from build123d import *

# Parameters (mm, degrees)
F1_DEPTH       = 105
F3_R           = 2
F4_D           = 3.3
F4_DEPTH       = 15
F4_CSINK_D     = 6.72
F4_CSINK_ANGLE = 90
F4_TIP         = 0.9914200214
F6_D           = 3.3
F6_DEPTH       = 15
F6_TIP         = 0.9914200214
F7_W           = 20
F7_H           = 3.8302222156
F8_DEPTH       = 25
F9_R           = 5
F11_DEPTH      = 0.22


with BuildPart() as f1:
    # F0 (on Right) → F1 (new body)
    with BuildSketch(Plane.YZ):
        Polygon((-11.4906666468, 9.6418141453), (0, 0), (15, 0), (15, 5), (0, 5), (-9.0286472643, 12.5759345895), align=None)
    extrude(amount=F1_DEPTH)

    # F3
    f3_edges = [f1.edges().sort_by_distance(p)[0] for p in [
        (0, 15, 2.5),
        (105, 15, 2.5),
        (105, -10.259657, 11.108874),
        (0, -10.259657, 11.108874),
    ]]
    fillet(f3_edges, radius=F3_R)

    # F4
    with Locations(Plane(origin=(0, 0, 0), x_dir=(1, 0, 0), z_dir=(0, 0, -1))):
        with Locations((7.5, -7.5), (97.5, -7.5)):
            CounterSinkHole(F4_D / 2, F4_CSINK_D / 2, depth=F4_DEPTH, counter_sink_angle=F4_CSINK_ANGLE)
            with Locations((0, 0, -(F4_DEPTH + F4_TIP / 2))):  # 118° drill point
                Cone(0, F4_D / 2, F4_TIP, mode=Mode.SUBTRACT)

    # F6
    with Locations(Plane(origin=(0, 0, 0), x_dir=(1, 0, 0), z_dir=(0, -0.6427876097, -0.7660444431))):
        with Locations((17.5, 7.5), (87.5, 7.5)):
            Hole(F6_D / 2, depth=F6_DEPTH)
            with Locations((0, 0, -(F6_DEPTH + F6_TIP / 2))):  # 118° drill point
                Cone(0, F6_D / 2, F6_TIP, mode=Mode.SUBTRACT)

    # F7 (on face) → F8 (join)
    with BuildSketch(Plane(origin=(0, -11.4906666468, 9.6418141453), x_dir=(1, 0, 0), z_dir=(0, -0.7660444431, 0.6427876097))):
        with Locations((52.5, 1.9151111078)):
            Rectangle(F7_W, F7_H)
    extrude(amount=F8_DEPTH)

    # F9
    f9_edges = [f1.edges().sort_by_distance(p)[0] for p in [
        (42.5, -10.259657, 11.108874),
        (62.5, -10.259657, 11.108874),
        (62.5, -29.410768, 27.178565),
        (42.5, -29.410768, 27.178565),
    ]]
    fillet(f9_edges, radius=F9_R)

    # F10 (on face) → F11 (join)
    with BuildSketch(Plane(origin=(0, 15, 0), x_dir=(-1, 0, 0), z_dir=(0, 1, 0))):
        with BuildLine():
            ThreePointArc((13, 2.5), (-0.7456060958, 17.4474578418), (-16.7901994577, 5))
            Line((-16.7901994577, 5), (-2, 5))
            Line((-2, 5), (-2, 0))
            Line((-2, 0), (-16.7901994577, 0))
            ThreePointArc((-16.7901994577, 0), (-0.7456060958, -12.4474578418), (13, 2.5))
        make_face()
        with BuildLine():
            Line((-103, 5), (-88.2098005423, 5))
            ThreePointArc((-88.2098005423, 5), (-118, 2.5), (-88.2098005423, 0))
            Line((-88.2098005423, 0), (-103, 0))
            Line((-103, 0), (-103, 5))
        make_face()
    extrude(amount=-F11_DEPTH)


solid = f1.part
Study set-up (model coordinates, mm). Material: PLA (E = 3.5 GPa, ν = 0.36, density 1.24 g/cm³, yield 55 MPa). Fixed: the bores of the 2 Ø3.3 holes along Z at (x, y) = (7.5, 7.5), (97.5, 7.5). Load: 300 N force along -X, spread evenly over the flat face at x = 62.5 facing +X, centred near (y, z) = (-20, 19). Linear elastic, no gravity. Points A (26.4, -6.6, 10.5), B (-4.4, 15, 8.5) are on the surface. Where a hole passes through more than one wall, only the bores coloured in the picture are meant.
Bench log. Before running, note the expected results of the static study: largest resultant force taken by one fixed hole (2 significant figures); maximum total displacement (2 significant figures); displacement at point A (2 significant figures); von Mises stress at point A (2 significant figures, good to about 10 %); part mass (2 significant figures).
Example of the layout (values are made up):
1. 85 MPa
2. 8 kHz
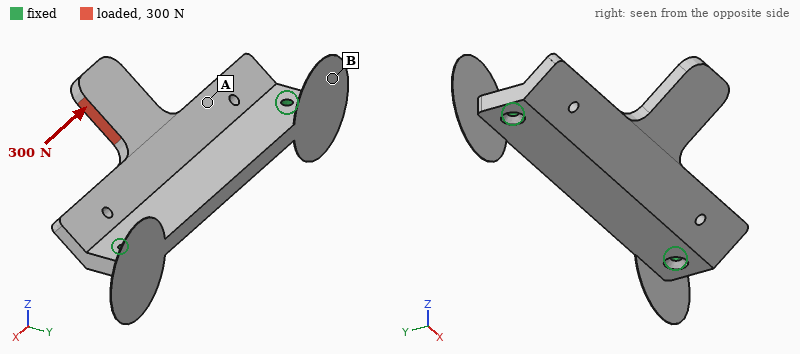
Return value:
1. 180 N
2. 0.30 mm
3. 0.11 mm
4. 6.0 MPa
5. 19 g
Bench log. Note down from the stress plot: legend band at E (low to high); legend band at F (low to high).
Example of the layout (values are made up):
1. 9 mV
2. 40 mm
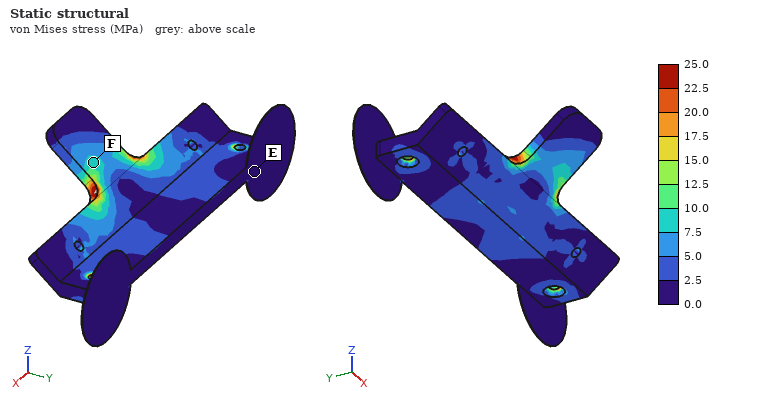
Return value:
1. 0.0 to 2.5 MPa
2. 7.5 to 10.0 MPa
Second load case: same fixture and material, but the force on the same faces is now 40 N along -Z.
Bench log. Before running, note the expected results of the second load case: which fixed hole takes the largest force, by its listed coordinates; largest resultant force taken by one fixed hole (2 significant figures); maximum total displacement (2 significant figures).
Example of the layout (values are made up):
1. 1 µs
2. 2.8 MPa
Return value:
1. (97.5, 7.5)
2. 26 N
3. 1.5 mm
